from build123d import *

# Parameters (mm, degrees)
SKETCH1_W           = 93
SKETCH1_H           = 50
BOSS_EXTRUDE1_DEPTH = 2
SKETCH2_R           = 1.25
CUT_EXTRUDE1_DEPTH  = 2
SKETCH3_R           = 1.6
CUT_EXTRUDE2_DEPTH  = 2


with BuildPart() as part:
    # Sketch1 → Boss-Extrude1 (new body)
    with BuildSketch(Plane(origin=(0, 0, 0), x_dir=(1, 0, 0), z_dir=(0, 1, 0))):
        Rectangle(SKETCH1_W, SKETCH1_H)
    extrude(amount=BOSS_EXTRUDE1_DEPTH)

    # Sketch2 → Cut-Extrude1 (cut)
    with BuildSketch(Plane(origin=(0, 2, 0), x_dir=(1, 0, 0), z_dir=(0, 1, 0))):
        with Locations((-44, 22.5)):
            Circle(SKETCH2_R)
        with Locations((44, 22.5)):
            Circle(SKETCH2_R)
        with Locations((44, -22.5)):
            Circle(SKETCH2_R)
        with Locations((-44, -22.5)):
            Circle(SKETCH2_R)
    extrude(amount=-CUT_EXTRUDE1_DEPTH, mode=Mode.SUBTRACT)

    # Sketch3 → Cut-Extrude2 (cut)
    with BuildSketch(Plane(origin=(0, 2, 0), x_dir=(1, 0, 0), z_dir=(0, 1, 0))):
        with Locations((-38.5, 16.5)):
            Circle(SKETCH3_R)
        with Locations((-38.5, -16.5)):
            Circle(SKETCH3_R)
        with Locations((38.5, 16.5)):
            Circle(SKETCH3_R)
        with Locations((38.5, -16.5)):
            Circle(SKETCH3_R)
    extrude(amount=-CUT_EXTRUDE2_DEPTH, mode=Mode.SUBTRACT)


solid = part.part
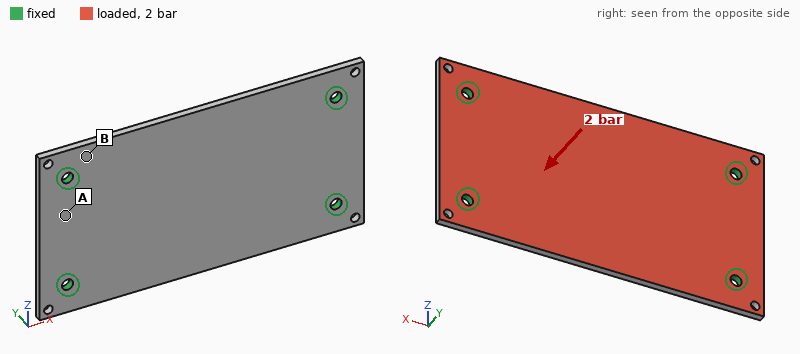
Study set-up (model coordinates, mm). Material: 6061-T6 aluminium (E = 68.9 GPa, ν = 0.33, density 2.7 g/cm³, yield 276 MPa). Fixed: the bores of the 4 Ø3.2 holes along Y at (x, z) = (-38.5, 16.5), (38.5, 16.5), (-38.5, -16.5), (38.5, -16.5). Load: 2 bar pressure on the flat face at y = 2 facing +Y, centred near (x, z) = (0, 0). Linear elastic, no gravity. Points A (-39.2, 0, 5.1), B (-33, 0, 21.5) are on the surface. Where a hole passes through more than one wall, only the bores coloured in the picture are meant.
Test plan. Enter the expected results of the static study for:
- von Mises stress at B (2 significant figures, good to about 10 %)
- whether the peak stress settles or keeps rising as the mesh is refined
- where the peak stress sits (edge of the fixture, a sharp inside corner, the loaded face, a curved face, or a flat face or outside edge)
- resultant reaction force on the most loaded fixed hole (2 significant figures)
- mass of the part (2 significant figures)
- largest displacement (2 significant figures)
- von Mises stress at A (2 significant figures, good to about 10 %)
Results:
98 MPa
keeps rising
edge of the fixture
230 N
25 g
0.45 mm
42 MPa
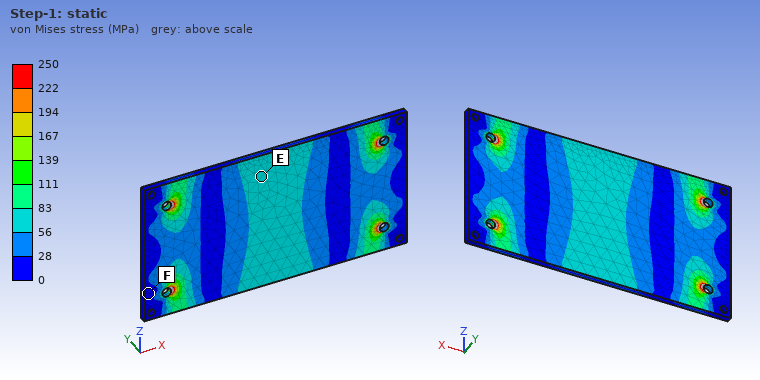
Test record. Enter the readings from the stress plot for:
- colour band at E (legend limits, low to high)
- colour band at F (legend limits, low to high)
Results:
56 to 83 MPa
0 to 28 MPa
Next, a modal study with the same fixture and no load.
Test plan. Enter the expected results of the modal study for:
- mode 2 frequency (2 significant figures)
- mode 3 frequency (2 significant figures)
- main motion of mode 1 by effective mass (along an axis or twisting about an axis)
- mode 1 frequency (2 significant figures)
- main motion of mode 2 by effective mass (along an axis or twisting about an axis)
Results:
2500 Hz
4600 Hz
along Y
1700 Hz
twisting about X
